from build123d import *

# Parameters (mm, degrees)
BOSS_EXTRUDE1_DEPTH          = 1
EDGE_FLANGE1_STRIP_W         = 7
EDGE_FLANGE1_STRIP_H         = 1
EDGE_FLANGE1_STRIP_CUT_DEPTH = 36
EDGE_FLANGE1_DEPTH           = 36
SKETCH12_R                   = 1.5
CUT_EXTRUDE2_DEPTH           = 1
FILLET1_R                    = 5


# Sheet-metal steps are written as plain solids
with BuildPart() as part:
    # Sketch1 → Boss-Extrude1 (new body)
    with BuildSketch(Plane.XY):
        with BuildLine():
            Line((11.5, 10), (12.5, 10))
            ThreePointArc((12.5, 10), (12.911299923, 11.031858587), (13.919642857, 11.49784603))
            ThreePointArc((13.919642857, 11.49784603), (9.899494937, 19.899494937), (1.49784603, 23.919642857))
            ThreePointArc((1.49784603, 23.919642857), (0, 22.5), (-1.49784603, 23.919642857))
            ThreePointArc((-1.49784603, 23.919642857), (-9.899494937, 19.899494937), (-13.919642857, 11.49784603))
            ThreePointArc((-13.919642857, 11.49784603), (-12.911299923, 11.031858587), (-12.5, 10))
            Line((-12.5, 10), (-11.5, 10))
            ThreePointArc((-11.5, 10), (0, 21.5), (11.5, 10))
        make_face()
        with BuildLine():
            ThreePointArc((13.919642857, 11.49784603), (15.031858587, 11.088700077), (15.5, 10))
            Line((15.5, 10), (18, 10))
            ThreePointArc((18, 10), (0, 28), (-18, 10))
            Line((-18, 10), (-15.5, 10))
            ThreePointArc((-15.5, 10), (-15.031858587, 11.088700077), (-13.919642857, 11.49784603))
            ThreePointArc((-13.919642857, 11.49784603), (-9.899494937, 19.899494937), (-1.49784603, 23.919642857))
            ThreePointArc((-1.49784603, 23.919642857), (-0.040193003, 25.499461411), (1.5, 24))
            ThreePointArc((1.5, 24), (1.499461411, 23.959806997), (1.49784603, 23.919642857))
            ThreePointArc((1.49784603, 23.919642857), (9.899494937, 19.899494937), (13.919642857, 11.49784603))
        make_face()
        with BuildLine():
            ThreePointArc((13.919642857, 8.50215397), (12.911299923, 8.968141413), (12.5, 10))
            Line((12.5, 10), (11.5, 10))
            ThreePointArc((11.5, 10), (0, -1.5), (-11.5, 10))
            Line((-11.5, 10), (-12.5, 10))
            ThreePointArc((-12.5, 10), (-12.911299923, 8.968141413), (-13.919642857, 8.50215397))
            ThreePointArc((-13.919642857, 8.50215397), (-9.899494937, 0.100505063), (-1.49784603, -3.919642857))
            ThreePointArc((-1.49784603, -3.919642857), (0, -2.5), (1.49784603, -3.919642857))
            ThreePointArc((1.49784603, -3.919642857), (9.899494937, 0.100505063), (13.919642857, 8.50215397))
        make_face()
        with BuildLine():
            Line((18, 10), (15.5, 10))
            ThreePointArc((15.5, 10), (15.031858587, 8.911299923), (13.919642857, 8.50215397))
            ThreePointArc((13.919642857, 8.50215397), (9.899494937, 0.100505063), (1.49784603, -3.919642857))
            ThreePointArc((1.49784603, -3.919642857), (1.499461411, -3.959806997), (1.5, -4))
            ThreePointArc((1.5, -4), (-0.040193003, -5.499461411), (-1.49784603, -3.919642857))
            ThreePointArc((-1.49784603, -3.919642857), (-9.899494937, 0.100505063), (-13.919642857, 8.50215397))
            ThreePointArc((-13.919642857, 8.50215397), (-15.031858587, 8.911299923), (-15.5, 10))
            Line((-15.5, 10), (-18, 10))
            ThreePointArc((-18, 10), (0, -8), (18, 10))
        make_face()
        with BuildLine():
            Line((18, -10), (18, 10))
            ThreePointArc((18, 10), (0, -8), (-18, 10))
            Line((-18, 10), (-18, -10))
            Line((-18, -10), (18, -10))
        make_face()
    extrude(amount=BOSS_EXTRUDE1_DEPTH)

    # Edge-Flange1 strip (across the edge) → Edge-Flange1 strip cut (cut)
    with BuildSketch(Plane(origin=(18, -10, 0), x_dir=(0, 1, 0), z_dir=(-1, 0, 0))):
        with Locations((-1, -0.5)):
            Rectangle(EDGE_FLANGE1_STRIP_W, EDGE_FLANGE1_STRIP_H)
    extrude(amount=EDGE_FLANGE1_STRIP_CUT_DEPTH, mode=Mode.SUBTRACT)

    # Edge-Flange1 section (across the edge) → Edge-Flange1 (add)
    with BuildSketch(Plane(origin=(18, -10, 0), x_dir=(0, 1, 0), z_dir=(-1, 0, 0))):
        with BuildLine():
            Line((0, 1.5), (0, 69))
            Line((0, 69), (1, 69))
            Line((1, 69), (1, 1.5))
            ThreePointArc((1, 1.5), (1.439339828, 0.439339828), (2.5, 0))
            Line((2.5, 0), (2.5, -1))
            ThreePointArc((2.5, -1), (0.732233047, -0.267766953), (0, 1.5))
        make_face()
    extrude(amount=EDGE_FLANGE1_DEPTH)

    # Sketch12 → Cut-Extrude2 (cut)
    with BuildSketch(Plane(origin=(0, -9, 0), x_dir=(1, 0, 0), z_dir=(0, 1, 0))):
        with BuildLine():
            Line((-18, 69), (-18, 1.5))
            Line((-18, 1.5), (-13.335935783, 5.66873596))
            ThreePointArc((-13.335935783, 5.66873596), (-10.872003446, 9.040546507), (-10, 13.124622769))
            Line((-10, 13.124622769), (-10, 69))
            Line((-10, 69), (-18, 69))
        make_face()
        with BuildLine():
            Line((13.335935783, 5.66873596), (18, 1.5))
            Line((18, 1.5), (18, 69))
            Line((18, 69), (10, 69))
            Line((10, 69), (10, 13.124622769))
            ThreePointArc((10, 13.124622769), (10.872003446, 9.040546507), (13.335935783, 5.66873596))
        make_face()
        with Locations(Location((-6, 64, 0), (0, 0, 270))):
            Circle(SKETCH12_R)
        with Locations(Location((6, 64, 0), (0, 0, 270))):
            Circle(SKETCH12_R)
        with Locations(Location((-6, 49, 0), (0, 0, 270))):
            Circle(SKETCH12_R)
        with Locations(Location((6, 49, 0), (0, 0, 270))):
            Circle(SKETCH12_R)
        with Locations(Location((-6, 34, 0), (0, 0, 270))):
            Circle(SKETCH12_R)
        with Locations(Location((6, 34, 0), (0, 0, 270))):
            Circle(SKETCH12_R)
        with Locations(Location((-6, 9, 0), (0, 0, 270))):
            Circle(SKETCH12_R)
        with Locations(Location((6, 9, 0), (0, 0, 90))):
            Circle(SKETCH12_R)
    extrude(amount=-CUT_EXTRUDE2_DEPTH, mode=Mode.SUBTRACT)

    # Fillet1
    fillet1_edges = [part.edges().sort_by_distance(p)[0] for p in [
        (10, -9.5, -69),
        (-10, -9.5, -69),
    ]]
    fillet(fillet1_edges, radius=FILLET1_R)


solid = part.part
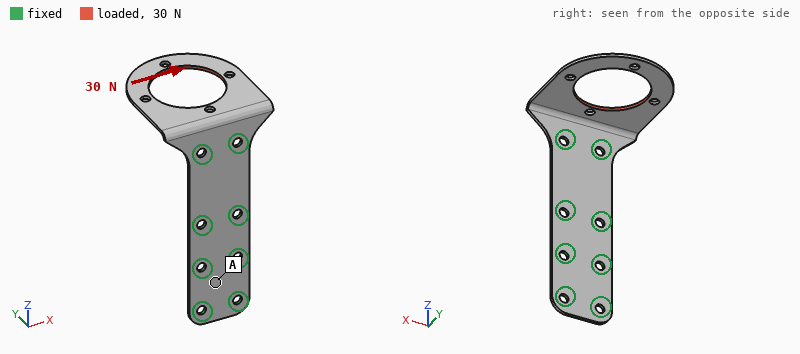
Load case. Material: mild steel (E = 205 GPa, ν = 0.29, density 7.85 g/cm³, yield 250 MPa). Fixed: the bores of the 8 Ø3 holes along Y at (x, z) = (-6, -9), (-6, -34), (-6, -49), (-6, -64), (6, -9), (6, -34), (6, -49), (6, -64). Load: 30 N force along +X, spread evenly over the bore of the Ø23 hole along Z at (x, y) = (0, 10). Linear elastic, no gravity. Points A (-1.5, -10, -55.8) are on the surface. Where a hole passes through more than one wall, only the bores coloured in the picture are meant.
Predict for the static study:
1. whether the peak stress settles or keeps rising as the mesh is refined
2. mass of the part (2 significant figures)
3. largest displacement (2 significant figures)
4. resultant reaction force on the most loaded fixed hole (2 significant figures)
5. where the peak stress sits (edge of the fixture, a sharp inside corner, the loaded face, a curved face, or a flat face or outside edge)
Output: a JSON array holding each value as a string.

["keeps rising", "17 g", "97 µm", "45 N", "edge of the fixture"]
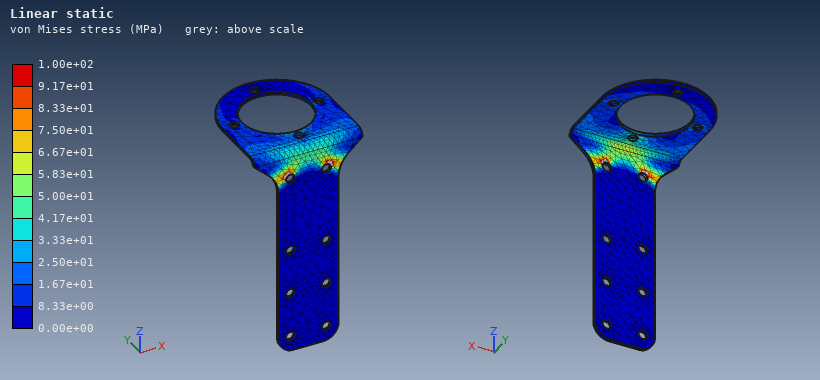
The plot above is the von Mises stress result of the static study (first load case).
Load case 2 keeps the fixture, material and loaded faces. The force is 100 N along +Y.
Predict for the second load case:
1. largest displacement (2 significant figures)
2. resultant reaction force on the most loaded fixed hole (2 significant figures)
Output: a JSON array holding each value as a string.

["0.32 mm", "50 N"]
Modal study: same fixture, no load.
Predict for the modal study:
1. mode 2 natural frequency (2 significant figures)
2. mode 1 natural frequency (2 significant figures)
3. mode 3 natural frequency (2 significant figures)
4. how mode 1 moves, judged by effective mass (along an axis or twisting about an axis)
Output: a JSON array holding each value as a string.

["1200 Hz", "520 Hz", "1800 Hz", "along Z"]
